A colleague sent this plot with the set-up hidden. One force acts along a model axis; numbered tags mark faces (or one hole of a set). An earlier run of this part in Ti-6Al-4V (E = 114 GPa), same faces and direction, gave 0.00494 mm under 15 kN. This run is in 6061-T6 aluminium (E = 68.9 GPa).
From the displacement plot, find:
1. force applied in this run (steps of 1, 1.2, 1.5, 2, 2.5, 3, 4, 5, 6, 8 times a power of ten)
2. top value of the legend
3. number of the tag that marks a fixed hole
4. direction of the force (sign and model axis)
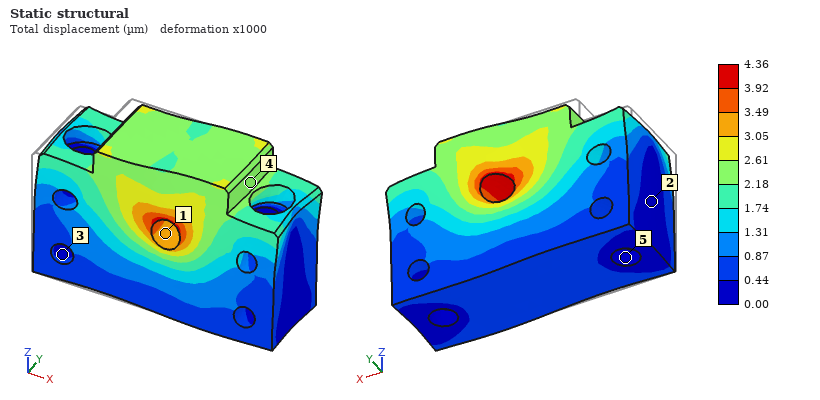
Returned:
8 kN
4.36 µm
5
+X
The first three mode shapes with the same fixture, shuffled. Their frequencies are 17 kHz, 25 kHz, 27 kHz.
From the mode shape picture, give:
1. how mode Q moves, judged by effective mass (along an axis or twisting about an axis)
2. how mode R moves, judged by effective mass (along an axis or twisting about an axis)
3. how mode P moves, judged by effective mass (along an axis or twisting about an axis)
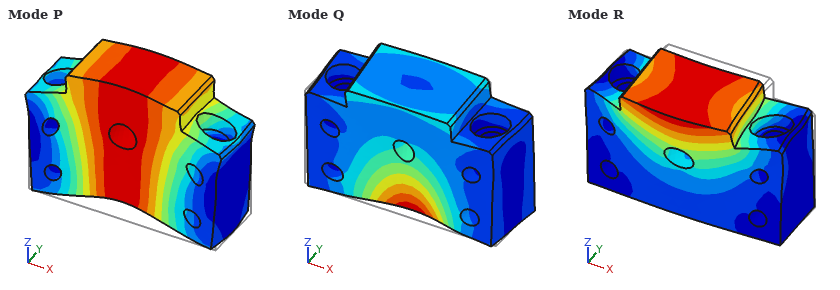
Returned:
along Y
along Y
along Z
